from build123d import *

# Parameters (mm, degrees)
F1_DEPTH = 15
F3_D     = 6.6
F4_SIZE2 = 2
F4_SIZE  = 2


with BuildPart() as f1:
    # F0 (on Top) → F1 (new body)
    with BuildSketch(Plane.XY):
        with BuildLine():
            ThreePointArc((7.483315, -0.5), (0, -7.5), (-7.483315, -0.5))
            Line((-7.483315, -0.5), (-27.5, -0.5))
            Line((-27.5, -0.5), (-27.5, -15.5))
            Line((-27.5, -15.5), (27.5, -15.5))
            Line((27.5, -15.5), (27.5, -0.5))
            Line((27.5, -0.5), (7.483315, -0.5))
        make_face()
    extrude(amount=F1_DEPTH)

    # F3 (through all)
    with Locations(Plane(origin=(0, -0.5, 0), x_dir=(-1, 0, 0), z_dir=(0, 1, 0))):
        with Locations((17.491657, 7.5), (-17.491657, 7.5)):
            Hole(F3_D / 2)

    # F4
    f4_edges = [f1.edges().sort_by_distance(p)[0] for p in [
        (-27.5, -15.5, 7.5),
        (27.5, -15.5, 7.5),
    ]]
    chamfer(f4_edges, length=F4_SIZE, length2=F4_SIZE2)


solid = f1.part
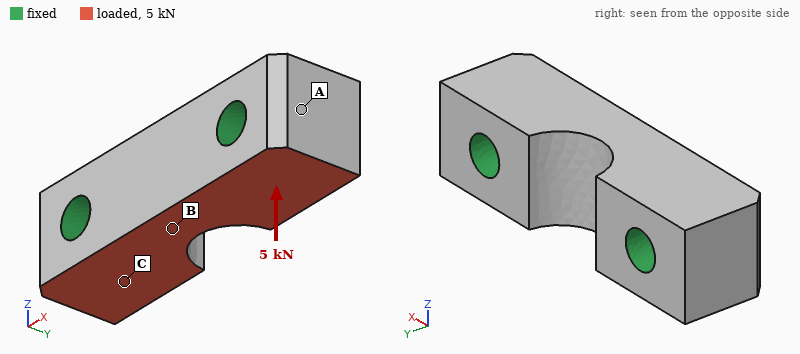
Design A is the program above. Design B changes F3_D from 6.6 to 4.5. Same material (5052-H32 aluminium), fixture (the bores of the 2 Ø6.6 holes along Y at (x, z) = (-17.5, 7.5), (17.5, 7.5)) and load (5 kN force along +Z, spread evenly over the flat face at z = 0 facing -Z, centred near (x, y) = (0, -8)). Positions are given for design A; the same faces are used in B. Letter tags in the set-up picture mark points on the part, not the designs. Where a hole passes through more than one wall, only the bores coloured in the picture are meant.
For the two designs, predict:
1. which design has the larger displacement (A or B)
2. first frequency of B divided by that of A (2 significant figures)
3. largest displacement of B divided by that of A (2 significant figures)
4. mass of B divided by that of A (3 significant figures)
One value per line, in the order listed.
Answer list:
B
0.80
1.2
1.05
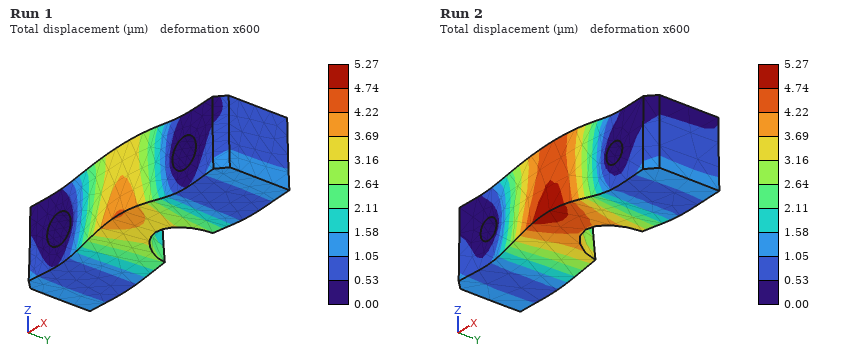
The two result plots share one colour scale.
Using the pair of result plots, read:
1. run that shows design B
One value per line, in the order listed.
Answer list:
Run 2
